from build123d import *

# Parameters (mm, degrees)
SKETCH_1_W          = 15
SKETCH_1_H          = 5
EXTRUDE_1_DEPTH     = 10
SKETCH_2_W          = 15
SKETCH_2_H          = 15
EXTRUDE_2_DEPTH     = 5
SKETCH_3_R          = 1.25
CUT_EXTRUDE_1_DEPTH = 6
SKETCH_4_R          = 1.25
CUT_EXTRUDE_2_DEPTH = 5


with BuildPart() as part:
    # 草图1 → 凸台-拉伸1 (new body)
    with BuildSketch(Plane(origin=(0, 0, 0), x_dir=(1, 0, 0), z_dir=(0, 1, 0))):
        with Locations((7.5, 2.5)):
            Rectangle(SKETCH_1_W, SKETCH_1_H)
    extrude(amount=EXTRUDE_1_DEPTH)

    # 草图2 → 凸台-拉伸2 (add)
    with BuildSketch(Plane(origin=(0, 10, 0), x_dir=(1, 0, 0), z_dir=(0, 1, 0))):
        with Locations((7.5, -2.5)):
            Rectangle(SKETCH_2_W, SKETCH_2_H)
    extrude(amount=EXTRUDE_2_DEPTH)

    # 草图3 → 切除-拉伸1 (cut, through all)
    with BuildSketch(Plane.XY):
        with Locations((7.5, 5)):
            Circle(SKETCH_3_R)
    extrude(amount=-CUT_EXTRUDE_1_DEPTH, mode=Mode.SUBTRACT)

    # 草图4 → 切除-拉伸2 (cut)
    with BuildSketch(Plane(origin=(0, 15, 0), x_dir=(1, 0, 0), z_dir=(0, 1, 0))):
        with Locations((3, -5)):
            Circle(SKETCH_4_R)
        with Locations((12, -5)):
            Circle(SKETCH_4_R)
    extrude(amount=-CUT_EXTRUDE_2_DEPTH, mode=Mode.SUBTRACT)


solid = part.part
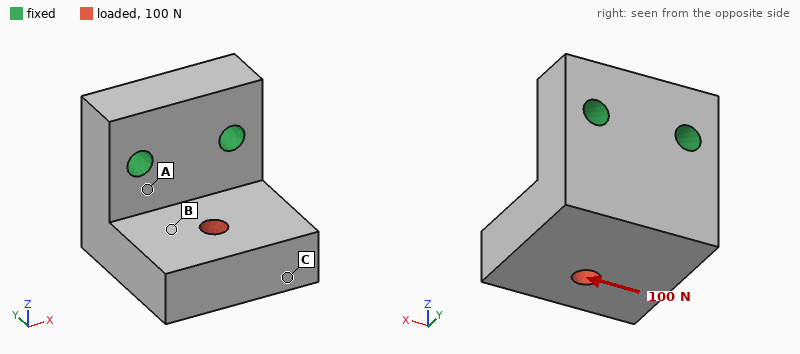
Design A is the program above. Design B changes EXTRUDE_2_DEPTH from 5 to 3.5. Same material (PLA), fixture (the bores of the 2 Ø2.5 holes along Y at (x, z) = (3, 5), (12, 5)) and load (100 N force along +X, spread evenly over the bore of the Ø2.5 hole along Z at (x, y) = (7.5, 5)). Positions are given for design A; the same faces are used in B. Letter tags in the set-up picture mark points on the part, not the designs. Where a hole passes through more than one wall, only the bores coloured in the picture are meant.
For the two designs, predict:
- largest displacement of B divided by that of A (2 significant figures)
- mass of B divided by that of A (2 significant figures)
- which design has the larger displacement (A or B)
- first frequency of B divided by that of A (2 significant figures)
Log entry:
1.5
0.82
B
0.70
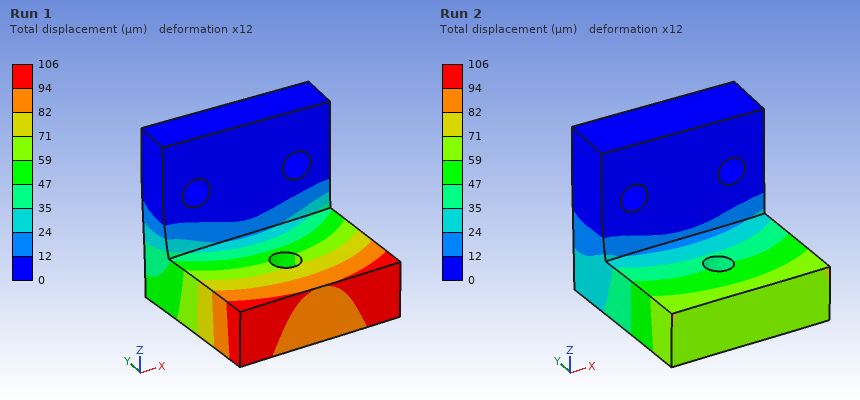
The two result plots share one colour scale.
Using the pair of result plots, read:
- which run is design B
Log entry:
Run 1
